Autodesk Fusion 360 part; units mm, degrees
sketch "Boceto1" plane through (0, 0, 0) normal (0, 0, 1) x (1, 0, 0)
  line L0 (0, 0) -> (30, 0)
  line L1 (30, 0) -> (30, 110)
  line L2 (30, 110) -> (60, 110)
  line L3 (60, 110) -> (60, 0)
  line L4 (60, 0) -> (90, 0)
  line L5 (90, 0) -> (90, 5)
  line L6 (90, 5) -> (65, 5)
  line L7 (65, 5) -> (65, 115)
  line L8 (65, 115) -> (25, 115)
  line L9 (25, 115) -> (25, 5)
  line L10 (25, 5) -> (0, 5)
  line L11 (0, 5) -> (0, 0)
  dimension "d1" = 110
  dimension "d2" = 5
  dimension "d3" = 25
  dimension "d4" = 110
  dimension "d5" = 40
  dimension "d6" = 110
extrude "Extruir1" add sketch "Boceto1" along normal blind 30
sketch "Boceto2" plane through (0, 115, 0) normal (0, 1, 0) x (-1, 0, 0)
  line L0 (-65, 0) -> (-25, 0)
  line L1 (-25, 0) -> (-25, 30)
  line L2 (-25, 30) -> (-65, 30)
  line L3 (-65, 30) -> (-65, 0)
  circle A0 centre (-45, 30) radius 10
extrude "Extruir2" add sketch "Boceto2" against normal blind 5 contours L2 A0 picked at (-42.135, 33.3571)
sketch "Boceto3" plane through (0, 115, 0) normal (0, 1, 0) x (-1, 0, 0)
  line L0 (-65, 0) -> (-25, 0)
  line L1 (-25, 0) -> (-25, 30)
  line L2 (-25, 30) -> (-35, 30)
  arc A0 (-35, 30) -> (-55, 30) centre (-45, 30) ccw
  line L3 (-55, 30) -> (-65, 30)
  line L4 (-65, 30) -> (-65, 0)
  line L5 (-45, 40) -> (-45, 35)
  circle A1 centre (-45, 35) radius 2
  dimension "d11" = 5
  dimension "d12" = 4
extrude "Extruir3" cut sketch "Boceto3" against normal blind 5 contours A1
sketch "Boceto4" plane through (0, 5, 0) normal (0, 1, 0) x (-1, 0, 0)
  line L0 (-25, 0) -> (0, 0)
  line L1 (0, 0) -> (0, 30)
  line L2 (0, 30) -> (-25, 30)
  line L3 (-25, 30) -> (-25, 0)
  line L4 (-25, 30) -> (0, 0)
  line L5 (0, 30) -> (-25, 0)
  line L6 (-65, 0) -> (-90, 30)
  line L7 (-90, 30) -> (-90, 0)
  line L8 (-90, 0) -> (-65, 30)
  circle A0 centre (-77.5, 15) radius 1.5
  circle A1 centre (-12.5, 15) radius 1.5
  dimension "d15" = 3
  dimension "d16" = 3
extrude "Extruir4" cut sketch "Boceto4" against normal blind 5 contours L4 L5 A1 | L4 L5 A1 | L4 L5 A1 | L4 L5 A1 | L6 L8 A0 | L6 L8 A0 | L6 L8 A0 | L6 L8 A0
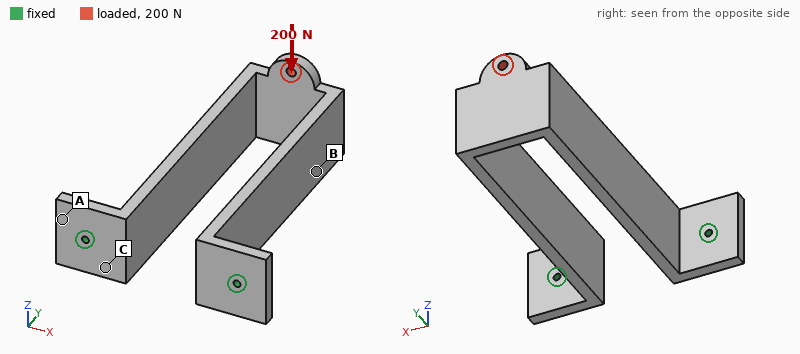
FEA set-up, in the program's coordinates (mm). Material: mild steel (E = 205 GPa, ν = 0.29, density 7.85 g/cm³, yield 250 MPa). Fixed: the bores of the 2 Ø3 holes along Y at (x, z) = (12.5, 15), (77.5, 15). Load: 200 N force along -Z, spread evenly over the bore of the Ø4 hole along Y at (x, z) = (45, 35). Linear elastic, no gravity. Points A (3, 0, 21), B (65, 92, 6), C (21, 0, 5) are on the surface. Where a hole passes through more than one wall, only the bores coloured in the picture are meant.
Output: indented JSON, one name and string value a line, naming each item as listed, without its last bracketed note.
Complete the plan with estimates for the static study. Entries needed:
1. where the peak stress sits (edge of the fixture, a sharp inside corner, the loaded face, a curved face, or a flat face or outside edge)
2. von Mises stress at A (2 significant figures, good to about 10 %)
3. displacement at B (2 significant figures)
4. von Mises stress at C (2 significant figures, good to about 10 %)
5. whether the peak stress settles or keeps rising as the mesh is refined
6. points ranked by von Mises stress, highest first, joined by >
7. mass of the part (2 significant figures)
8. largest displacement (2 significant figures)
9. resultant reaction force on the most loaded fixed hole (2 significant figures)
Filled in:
{
  "where the peak stress sits": "edge of the fixture",
  "von Mises stress at A": "24 MPa",
  "displacement at B": "0.19 mm",
  "von Mises stress at C": "36 MPa",
  "whether the peak stress settles or keeps rising as the mesh is refined": "keeps rising",
  "points ranked by von Mises stress, highest first, joined by >": "C > A > B",
  "mass of the part": "370 g",
  "largest displacement": "0.25 mm",
  "resultant reaction force on the most loaded fixed hole": "100 N"
}
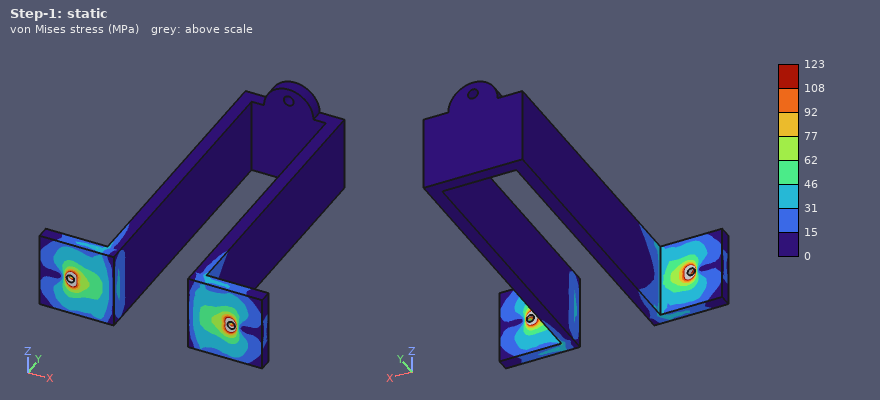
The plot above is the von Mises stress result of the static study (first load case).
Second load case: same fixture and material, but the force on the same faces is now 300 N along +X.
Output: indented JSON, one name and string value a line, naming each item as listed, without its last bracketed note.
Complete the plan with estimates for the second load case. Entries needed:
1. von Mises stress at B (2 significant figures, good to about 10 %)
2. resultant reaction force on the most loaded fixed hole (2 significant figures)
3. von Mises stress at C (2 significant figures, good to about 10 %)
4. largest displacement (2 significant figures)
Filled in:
{
  "von Mises stress at B": "43 MPa",
  "resultant reaction force on the most loaded fixed hole": "510 N",
  "von Mises stress at C": "34 MPa",
  "largest displacement": "0.38 mm"
}
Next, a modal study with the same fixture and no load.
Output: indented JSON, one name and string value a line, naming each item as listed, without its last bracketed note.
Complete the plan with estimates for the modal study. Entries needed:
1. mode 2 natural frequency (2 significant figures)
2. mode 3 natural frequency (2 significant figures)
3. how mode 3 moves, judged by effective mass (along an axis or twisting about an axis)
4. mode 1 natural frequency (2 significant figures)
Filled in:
{
  "mode 2 natural frequency": "400 Hz",
  "mode 3 natural frequency": "1100 Hz",
  "how mode 3 moves, judged by effective mass": "twisting about Y",
  "mode 1 natural frequency": "400 Hz"
}
